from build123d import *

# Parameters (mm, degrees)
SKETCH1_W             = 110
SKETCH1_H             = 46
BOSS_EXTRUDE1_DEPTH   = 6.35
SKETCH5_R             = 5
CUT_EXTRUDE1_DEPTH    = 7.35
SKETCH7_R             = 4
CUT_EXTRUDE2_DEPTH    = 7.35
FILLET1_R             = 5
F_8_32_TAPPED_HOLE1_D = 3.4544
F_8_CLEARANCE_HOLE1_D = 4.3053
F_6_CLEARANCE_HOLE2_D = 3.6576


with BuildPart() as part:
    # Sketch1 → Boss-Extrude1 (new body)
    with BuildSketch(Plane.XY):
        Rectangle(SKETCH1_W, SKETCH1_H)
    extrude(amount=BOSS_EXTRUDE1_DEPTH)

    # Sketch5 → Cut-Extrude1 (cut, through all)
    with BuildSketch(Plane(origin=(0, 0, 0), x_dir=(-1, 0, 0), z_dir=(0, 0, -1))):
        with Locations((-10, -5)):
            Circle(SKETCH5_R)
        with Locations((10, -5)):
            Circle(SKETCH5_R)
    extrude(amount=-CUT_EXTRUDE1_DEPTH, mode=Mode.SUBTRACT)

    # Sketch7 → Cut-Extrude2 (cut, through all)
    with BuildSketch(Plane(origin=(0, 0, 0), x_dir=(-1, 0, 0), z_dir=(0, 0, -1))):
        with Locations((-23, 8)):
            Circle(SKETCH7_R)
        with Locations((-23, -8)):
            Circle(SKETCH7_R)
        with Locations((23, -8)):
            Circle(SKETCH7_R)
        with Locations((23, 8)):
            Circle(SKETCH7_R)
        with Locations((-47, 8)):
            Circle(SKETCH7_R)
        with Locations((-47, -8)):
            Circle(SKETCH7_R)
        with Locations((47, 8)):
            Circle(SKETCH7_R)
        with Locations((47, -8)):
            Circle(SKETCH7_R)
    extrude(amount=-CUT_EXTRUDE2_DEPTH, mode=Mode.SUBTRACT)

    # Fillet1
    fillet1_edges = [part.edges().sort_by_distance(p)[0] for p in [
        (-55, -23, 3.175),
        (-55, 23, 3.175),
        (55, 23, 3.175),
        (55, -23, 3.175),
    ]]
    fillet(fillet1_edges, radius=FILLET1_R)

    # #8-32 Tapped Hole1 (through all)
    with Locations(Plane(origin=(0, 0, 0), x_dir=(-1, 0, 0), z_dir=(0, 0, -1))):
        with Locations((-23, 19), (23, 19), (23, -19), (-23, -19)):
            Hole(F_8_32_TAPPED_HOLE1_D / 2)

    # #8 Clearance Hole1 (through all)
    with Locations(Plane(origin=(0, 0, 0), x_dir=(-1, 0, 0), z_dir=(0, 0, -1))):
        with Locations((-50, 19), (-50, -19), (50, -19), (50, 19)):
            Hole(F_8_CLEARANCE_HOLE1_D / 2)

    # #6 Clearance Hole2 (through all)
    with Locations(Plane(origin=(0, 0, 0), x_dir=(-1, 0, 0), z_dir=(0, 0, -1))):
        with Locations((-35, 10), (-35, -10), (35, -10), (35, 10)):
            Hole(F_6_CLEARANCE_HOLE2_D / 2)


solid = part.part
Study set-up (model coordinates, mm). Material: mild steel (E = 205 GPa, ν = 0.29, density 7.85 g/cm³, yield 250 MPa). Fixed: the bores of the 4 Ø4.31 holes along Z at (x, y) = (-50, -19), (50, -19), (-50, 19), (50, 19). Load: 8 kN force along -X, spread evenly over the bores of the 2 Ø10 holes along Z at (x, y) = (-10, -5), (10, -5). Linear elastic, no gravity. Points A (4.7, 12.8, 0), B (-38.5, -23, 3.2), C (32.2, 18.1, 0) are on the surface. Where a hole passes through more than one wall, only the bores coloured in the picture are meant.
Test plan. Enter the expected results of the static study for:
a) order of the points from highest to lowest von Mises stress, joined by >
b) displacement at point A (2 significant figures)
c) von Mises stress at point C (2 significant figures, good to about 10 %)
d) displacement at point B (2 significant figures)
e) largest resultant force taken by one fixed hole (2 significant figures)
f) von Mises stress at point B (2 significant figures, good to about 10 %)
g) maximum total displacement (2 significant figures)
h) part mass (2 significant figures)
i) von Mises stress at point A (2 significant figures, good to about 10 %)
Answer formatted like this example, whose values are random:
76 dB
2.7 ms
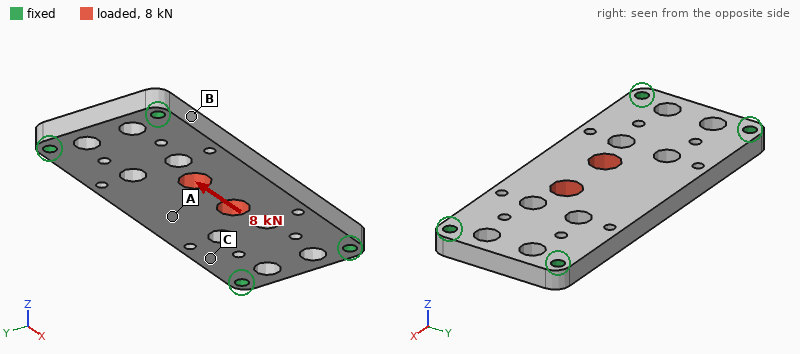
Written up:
B > C > A
3.5 µm
15 MPa
1.5 µm
2.2 kN
30 MPa
6.8 µm
220 g
6.7 MPa
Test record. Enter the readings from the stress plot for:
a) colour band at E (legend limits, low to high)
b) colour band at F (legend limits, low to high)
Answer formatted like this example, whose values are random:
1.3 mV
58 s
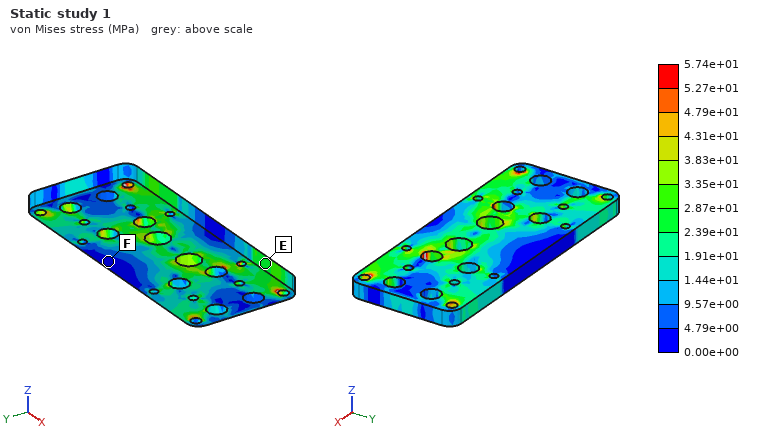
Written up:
2.39e+01 to 2.87e+01 MPa
0.00e+00 to 4.79e+00 MPa
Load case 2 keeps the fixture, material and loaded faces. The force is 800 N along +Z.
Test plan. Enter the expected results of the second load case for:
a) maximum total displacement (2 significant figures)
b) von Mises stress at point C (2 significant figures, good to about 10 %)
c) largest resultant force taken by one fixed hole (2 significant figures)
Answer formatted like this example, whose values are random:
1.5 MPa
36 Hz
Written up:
30 µm
7.0 MPa
250 N
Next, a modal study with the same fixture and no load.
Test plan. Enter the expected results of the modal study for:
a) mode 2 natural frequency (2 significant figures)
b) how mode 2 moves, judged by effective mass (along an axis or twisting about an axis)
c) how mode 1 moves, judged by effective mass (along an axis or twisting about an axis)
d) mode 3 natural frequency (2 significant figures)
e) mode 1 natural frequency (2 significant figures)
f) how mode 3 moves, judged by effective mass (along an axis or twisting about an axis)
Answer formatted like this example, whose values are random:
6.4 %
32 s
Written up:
5200 Hz
twisting about X
along Z
7600 Hz
2900 Hz
twisting about Y
